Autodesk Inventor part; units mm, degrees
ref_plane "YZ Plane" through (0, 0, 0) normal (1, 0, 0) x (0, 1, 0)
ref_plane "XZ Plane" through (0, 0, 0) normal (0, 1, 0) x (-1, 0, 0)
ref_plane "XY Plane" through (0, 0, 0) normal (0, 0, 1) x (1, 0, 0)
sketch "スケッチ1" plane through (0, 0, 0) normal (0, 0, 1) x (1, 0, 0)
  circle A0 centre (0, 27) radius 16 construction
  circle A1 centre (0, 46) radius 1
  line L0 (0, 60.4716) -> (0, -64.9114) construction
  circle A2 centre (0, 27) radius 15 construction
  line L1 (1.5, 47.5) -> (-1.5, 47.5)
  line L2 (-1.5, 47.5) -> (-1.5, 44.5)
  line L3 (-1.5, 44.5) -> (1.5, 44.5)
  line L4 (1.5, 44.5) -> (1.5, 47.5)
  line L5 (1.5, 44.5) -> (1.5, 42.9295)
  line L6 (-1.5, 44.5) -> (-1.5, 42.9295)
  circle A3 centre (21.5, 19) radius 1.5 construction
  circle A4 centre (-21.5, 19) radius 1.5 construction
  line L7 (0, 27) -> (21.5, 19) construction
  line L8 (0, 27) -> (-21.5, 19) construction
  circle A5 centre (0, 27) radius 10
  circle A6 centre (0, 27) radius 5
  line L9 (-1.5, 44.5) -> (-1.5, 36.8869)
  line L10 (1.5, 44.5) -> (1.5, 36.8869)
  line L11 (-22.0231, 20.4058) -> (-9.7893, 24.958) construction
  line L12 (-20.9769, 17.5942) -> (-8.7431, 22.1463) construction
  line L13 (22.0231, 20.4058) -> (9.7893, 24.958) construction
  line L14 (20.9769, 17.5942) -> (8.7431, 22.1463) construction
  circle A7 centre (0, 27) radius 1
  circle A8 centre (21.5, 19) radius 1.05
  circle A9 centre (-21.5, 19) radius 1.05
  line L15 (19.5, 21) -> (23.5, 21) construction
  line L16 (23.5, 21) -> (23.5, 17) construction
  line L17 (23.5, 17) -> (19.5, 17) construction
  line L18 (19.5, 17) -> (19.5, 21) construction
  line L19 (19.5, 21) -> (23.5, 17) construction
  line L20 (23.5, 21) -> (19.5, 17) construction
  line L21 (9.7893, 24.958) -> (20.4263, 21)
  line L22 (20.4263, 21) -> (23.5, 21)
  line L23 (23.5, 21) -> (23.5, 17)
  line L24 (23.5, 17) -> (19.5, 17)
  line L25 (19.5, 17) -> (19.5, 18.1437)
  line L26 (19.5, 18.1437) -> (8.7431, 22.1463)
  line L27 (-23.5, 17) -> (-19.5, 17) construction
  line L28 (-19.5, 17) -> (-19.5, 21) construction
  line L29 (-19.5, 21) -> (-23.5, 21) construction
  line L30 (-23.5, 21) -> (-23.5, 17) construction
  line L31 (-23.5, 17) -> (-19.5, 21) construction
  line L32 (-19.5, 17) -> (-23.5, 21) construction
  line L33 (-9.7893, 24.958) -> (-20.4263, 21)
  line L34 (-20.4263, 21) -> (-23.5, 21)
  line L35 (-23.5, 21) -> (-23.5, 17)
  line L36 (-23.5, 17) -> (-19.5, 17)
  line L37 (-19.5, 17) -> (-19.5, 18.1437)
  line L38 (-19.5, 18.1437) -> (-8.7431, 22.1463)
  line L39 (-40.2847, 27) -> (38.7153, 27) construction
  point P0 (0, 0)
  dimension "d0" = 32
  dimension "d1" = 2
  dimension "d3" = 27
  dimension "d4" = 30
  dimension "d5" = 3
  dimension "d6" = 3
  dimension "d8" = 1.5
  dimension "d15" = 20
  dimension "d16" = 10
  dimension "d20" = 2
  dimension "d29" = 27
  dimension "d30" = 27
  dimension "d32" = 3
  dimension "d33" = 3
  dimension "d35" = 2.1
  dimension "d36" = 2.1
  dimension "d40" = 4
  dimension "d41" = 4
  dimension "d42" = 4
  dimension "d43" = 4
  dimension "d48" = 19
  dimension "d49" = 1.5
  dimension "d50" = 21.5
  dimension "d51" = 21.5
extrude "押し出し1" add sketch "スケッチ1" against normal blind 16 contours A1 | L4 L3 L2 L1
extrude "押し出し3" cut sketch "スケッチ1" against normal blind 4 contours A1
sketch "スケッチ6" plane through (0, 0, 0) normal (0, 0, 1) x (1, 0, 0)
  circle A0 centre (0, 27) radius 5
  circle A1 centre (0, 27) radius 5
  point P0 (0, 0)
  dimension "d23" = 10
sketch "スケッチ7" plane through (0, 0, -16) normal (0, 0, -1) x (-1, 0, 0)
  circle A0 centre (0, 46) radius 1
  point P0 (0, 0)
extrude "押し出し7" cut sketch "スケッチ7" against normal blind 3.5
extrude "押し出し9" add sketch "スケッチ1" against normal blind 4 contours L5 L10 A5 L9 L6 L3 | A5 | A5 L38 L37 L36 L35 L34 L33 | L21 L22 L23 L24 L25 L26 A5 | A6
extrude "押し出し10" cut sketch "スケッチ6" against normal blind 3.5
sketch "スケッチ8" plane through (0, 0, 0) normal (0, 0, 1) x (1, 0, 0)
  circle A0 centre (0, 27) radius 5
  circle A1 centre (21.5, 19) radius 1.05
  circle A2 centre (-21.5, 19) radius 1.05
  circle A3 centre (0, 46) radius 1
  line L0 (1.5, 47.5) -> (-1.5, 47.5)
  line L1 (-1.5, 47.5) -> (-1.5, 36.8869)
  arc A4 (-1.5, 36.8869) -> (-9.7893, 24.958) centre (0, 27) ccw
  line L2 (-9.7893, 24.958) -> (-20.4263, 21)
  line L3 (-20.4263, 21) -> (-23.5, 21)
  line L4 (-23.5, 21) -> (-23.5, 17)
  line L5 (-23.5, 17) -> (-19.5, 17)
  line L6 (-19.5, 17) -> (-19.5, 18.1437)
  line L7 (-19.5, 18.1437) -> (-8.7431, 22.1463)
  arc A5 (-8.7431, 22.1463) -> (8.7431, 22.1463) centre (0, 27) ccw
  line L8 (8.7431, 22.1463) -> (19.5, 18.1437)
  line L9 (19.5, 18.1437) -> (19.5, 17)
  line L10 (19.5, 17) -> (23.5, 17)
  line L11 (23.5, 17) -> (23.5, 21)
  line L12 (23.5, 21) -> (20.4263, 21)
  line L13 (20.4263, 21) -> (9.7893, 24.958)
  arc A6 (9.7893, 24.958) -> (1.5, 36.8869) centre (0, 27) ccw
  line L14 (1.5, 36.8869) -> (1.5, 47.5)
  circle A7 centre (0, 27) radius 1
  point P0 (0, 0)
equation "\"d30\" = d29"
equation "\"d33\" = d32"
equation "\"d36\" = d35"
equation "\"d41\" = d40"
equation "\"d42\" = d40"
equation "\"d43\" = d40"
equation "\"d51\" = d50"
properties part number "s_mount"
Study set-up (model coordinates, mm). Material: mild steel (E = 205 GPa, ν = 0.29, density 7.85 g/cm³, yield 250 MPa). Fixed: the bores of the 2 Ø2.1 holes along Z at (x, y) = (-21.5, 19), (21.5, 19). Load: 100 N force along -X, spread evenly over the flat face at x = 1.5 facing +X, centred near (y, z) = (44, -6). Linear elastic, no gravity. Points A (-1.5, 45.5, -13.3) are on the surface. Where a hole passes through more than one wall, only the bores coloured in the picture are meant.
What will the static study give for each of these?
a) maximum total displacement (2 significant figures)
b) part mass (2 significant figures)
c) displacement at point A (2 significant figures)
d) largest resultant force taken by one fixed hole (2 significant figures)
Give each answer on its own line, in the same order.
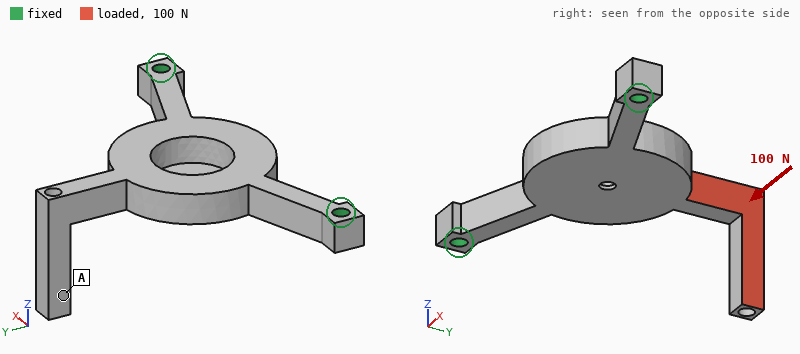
74 µm
12 g
59 µm
89 N
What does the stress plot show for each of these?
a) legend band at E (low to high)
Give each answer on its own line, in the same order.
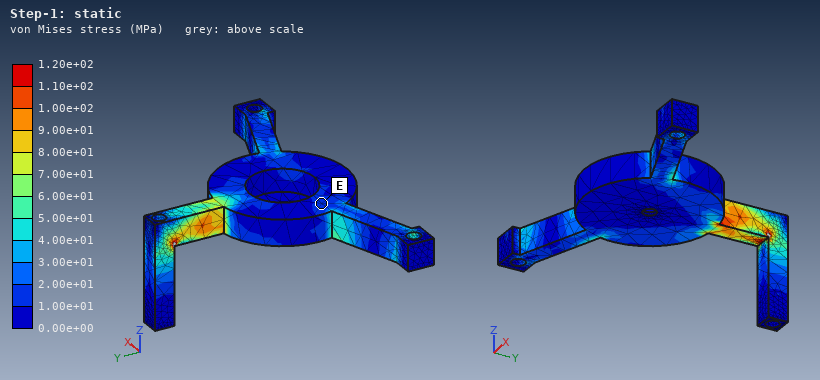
1.00e+01 to 2.00e+01 MPa
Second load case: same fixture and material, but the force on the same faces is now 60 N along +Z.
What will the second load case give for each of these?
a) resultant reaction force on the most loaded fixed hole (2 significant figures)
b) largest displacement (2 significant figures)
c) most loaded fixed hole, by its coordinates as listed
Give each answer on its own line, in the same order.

33 N
0.18 mm
(21.5, 19)
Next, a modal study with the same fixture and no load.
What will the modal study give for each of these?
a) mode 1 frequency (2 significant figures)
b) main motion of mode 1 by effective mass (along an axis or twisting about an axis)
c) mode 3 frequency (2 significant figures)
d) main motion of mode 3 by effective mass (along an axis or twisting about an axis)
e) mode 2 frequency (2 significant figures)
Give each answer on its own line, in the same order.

2100 Hz
along Z
7600 Hz
along Z
5900 Hz
